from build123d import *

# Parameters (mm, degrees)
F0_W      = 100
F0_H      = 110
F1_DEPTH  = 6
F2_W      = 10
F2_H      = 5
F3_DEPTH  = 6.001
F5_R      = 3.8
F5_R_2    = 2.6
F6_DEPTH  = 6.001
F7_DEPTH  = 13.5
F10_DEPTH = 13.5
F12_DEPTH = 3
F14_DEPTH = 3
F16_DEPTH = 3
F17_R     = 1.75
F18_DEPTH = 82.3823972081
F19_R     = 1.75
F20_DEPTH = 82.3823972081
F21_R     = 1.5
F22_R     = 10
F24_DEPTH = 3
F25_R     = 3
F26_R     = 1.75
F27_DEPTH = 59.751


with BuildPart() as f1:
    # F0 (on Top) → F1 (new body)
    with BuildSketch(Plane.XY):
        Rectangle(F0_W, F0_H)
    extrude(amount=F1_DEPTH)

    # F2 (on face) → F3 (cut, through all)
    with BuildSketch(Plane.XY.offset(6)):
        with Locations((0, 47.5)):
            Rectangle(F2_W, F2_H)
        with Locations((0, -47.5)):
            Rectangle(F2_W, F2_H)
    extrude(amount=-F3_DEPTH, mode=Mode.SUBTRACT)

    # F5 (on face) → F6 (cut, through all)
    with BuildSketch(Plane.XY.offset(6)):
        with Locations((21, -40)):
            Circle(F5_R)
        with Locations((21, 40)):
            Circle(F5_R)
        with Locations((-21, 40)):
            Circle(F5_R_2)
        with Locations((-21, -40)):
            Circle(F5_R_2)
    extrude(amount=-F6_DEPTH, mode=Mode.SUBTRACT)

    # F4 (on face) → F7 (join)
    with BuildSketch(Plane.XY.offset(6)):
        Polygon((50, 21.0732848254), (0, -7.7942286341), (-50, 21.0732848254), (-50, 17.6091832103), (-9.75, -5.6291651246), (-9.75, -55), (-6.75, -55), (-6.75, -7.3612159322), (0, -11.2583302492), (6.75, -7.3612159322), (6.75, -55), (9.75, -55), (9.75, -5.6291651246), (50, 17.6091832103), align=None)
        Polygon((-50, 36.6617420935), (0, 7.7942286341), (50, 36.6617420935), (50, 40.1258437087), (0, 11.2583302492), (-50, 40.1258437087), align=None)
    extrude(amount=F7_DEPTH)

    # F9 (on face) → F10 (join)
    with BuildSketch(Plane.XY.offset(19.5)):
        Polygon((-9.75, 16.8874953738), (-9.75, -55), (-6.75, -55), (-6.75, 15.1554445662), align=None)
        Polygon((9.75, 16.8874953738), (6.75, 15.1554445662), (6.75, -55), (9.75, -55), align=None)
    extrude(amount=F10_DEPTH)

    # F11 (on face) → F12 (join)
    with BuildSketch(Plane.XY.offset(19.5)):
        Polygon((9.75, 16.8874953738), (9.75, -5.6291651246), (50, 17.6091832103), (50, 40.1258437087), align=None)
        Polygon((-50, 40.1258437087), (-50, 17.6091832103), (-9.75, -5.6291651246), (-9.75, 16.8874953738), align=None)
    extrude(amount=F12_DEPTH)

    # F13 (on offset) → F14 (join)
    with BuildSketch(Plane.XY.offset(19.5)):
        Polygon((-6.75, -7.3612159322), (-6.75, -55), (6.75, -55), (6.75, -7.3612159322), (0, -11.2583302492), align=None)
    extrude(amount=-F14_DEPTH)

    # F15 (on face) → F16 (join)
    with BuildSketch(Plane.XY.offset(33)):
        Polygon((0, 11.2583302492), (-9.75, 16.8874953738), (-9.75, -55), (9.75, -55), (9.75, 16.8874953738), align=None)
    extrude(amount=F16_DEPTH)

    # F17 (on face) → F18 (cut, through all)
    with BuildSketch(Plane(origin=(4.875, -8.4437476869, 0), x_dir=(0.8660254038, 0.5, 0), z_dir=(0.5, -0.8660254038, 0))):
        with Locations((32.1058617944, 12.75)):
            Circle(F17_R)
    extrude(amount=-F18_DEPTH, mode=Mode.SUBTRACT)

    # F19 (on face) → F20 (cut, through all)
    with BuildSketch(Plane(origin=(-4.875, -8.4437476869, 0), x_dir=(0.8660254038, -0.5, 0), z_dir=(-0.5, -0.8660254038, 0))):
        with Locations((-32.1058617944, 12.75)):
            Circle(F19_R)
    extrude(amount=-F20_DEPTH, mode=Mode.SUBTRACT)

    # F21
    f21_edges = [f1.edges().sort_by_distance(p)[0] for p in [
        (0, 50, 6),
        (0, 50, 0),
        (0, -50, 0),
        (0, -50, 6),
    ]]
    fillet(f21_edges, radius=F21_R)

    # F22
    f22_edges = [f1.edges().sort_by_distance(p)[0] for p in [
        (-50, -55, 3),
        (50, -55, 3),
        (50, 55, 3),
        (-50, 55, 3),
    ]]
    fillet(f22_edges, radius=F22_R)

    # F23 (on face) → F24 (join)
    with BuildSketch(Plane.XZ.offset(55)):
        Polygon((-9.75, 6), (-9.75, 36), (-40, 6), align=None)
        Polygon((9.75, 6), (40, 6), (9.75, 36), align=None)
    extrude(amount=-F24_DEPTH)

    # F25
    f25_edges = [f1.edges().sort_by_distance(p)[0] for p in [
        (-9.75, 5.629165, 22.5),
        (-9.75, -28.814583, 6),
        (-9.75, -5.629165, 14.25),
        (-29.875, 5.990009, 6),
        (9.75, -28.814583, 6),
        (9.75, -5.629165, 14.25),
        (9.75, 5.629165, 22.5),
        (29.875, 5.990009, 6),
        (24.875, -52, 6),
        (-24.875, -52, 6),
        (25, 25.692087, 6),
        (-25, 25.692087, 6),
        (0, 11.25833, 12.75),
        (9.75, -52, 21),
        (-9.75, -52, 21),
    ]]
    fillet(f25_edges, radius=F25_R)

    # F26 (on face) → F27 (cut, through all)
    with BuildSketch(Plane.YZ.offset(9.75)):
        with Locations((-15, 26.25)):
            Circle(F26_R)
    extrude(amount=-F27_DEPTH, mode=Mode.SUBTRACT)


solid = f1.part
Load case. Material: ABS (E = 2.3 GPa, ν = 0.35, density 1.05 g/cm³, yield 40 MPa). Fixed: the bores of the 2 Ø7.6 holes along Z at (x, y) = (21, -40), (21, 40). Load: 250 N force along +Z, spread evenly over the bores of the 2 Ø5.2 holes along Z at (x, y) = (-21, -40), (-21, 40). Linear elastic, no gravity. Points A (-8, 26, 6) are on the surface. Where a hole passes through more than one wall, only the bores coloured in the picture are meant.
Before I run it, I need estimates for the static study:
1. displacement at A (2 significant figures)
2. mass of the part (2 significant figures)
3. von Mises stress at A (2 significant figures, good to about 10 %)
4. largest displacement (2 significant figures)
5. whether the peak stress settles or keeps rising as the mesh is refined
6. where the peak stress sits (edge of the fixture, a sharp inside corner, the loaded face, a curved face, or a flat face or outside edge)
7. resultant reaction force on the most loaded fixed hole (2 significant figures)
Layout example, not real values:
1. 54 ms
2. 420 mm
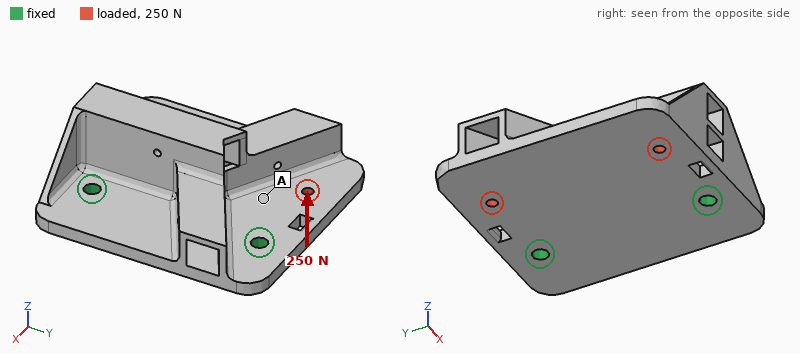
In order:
1. 0.59 mm
2. 100 g
3. 2.9 MPa
4. 1.6 mm
5. keeps rising
6. edge of the fixture
7. 130 N
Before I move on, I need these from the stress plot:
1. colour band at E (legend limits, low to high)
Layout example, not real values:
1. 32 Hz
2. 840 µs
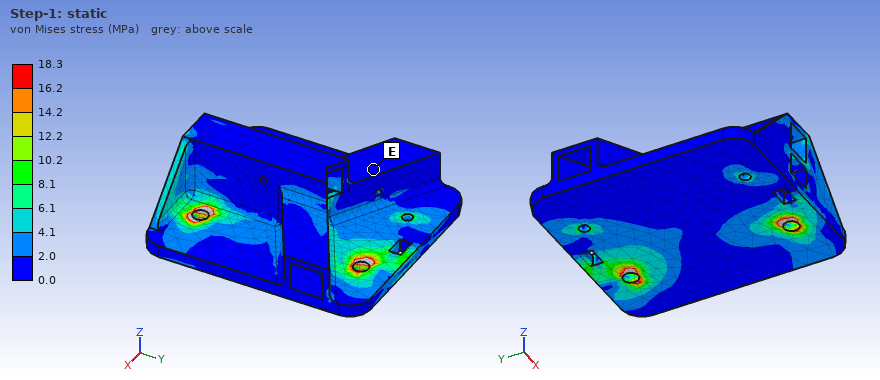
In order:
1. 0.0 to 2.0 MPa
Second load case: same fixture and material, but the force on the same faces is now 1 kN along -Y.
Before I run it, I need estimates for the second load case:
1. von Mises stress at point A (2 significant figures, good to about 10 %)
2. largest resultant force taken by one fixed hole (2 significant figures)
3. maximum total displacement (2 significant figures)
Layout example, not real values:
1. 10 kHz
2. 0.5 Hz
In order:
1. 3.3 MPa
2. 720 N
3. 0.20 mm
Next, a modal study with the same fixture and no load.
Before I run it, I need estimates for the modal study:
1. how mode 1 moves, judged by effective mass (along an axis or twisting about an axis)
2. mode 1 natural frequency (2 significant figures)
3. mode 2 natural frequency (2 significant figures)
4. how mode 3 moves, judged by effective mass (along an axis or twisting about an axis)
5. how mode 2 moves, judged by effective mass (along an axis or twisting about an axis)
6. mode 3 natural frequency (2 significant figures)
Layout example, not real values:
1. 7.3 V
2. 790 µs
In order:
1. along Z
2. 310 Hz
3. 930 Hz
4. along Z
5. twisting about X
6. 1300 Hz
